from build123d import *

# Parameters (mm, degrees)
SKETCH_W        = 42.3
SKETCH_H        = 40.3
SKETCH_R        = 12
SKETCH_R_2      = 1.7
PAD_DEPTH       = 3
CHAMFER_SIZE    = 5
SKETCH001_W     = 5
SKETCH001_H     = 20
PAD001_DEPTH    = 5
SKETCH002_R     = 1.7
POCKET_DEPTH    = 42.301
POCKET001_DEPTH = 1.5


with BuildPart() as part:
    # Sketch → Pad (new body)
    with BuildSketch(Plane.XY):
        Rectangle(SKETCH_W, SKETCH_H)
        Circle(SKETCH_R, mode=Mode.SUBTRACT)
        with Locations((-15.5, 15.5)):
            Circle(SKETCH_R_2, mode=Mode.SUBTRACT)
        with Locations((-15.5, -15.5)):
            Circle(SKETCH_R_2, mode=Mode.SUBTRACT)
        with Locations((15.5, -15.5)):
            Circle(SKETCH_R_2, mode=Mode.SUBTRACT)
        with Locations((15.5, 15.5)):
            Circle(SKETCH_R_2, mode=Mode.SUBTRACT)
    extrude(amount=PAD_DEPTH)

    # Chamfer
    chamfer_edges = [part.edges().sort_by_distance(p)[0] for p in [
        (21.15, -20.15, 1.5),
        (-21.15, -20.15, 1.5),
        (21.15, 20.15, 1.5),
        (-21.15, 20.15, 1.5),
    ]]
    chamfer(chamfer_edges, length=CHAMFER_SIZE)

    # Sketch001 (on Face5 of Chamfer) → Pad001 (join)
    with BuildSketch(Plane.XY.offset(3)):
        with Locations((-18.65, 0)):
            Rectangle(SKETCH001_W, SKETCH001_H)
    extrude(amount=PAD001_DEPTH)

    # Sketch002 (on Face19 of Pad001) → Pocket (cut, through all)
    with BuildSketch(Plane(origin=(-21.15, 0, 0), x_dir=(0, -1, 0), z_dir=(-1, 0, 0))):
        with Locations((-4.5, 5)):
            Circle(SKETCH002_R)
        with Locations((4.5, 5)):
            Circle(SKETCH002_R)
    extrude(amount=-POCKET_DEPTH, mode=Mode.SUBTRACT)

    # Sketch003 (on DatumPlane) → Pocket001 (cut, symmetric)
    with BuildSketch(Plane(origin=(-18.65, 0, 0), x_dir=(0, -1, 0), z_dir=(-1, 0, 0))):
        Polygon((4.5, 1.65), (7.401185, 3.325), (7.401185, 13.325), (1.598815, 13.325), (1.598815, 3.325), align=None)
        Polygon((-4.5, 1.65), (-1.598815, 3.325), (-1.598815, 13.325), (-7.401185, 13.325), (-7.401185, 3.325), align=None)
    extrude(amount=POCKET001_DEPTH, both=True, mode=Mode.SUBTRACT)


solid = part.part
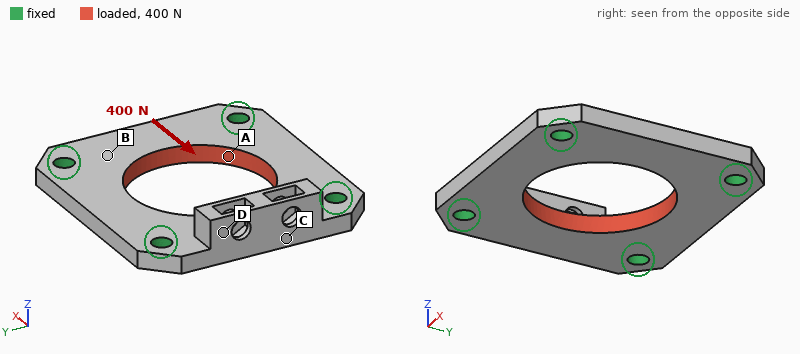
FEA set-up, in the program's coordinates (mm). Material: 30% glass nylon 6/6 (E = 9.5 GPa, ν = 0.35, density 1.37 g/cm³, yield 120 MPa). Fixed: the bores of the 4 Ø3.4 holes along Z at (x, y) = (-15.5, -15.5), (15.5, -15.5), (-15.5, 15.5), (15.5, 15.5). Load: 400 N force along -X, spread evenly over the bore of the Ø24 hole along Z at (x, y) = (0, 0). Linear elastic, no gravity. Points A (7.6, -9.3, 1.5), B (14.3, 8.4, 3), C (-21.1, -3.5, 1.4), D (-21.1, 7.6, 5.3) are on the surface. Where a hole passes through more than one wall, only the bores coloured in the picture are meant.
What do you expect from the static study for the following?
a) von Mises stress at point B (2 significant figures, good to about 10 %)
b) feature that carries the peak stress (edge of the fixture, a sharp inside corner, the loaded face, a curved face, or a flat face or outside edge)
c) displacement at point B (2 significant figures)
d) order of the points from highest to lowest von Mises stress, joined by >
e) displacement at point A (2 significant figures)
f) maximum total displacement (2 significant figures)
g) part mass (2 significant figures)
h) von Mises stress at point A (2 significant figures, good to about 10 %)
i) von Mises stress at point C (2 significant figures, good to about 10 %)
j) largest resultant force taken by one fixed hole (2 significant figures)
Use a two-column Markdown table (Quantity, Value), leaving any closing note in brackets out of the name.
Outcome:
| Quantity | Value |
|---|---|
| von Mises stress at point B | 2.7 MPa |
| feature that carries the peak stress | edge of the fixture |
| displacement at point B | 5.3 µm |
| order of the points from highest to lowest von Mises stress, joined by > | A > C > B > D |
| displacement at point A | 5.4 µm |
| maximum total displacement | 10 µm |
| part mass | 5.2 g |
| von Mises stress at point A | 4.9 MPa |
| von Mises stress at point C | 4.0 MPa |
| largest resultant force taken by one fixed hole | 100 N |
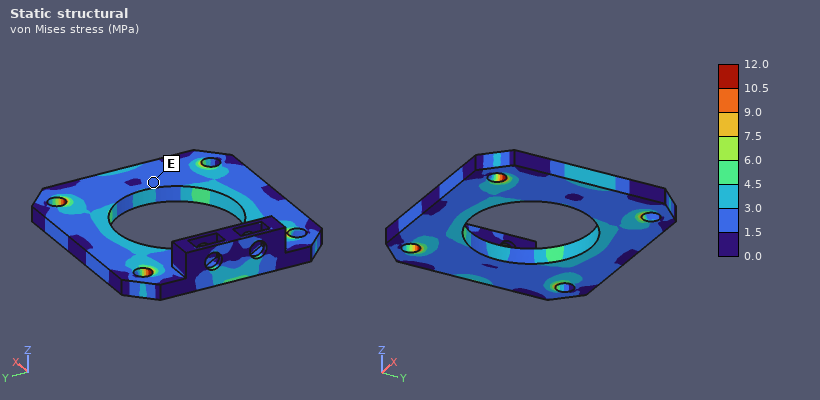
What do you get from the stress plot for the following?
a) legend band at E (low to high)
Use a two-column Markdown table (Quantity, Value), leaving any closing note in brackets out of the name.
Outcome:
| Quantity | Value |
|---|---|
| legend band at E | 1.5 to 3.0 MPa |
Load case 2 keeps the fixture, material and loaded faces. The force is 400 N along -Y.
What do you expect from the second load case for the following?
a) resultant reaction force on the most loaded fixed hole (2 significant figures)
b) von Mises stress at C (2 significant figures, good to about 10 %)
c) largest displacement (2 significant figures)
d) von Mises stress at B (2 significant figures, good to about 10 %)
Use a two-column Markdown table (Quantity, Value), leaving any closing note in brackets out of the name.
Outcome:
| Quantity | Value |
|---|---|
| resultant reaction force on the most loaded fixed hole | 100 N |
| von Mises stress at C | 1.2 MPa |
| largest displacement | 11 µm |
| von Mises stress at B | 3.0 MPa |
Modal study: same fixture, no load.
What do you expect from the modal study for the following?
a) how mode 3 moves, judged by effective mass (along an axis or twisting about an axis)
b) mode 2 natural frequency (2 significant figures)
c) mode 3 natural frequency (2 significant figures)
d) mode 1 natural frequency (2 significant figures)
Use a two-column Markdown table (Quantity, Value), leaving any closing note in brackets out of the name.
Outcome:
| Quantity | Value |
|---|---|
| how mode 3 moves, judged by effective mass | twisting about X |
| mode 2 natural frequency | 9000 Hz |
| mode 3 natural frequency | 9400 Hz |
| mode 1 natural frequency | 8900 Hz |
